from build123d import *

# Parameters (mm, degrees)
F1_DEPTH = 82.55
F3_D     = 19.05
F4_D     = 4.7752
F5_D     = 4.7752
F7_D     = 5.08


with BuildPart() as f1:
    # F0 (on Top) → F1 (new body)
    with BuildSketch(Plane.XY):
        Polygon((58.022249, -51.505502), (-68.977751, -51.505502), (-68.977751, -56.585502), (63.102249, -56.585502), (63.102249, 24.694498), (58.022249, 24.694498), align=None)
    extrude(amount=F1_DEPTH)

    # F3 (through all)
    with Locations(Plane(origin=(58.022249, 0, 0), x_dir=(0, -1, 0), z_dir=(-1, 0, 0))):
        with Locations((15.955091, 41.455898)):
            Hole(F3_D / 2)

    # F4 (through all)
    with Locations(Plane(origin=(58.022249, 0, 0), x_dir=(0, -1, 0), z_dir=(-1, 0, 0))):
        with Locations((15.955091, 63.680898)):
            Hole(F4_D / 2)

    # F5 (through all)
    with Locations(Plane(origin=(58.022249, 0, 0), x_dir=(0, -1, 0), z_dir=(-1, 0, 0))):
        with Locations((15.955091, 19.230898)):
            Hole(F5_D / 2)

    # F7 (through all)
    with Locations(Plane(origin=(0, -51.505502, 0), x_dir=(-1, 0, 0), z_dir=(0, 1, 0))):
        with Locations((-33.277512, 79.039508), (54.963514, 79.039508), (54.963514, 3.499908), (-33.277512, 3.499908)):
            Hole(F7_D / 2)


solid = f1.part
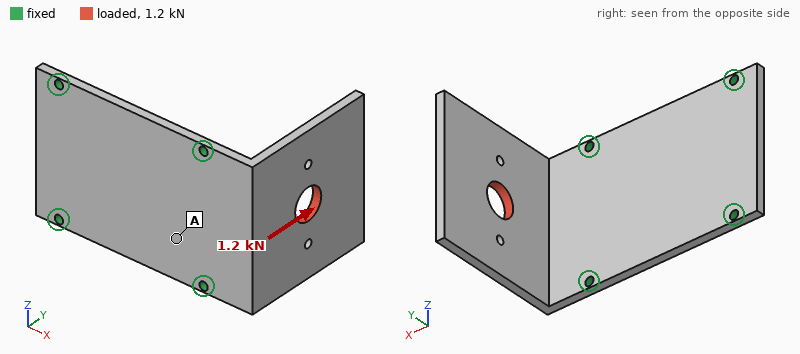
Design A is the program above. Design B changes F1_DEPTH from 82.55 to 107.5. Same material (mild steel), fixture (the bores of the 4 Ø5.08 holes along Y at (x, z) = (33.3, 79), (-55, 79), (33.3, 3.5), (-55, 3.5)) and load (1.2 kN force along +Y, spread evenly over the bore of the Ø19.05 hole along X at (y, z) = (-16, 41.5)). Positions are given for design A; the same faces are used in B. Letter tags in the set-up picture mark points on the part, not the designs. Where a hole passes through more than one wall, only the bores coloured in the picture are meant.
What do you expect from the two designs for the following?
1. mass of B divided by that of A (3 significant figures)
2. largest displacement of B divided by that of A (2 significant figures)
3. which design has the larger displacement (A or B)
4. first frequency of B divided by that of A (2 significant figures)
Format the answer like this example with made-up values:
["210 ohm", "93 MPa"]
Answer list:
["1.31", "0.83", "A", "1.0"]
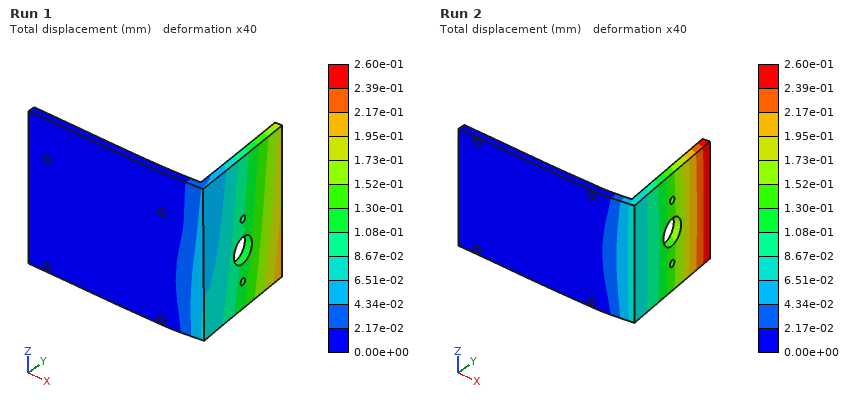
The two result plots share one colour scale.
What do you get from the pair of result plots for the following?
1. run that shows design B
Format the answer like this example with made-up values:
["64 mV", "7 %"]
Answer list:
["Run 1"]
